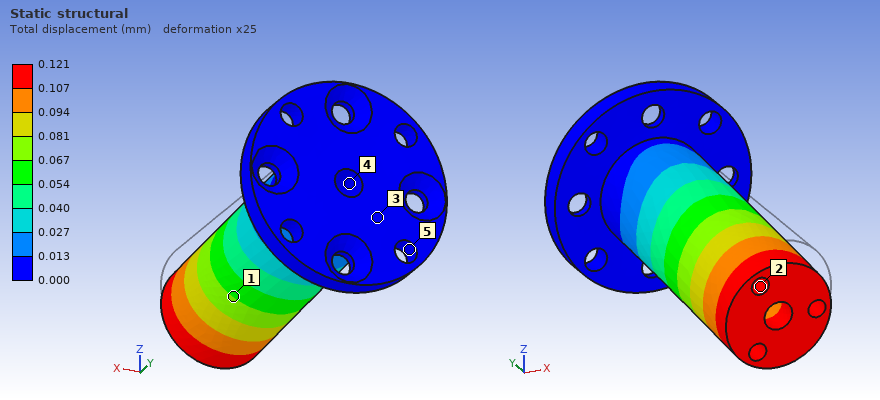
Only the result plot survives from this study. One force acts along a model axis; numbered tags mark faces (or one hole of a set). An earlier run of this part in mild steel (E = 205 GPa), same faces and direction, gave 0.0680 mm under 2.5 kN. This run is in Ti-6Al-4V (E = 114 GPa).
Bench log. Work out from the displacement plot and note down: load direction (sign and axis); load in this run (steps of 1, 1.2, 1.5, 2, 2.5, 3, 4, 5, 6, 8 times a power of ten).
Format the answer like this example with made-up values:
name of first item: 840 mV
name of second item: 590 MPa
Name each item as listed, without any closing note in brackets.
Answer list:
load direction: -Z
load in this run: 2.5 kN
